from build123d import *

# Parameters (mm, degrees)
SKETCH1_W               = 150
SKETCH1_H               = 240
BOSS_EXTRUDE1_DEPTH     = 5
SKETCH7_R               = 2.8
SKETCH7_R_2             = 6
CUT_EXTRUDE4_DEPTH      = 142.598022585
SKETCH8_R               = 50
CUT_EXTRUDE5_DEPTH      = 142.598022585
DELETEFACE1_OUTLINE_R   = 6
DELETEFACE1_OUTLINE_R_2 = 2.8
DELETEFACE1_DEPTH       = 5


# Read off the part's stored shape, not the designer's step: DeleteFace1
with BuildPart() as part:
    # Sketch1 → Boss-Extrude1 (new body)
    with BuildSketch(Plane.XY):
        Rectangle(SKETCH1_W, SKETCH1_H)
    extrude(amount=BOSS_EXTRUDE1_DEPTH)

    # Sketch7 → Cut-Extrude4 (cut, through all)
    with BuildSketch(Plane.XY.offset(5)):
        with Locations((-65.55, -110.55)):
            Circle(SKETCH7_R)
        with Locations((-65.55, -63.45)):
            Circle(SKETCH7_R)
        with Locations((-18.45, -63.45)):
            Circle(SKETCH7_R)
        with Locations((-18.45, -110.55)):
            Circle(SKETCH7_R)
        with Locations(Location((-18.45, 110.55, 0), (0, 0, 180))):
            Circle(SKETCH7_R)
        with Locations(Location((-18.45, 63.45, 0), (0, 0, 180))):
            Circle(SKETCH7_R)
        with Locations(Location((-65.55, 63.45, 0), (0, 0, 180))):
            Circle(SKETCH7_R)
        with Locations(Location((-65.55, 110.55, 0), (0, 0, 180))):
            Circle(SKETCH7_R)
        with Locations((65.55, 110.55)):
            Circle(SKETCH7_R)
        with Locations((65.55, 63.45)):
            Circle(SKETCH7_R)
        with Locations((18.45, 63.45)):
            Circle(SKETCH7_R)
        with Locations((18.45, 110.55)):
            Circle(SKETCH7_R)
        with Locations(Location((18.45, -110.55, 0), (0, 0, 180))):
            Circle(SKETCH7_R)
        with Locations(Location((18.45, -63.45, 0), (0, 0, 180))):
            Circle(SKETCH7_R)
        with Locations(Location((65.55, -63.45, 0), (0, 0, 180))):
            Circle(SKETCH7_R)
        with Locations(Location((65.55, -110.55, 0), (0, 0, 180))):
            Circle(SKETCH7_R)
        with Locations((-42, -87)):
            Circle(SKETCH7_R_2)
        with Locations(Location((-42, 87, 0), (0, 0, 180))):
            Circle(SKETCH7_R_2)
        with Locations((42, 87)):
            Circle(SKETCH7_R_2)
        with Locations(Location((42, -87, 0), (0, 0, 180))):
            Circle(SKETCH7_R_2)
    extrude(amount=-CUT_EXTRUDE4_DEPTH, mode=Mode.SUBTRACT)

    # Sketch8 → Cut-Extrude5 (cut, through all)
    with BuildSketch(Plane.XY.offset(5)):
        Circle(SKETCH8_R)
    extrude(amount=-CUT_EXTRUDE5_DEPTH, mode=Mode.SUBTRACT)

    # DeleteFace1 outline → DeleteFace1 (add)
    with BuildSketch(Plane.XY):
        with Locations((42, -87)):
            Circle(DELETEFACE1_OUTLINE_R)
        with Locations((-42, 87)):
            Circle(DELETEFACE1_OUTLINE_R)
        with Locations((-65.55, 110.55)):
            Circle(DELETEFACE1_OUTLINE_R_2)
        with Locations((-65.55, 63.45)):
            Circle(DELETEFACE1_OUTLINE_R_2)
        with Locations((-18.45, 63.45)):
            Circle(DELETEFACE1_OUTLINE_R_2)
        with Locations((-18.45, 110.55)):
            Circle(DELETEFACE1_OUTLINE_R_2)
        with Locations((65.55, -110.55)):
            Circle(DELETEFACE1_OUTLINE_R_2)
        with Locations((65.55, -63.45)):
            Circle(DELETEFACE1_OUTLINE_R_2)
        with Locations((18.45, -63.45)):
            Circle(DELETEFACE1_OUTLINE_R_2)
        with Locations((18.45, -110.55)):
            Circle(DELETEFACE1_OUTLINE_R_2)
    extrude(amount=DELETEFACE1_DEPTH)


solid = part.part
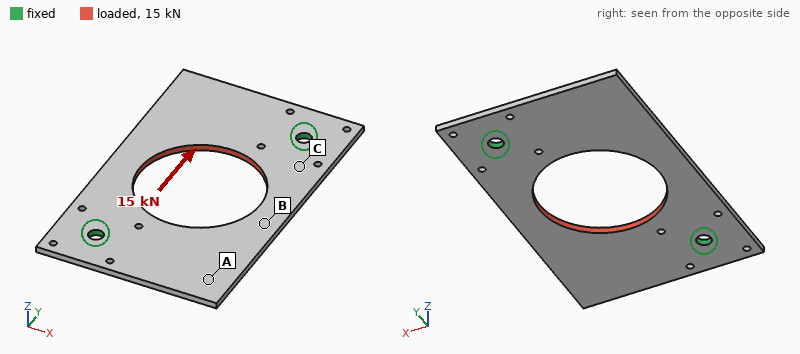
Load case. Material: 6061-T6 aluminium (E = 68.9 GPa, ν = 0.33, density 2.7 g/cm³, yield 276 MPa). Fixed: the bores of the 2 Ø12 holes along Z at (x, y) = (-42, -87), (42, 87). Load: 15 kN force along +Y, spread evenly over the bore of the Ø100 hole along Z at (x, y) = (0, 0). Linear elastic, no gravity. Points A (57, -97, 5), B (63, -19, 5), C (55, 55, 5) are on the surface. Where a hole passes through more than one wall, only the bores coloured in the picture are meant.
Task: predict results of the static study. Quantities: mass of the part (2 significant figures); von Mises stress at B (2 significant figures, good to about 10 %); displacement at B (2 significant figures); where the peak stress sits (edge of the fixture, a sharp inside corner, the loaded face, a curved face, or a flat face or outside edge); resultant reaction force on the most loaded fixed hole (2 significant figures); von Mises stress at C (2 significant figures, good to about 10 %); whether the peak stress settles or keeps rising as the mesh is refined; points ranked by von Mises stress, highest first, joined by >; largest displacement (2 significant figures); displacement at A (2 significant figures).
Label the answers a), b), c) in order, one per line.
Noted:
a) 370 g
b) 14 MPa
c) 37 µm
d) edge of the fixture
e) 7.5 kN
f) 28 MPa
g) keeps rising
h) C > B > A
i) 49 µm
j) 43 µm
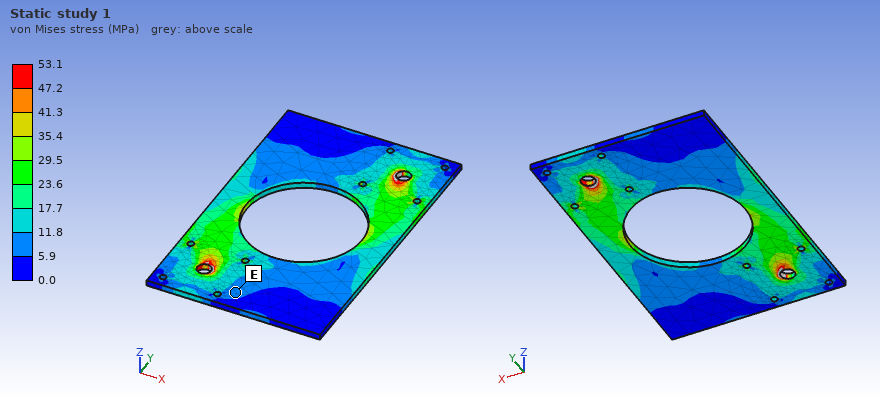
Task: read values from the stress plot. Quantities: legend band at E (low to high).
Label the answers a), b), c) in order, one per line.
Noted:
a) 5.9 to 11.8 MPa
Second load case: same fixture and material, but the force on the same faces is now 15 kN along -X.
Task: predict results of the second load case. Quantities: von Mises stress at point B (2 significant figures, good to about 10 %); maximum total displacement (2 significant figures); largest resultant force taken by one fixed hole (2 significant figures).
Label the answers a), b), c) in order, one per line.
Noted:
a) 26 MPa
b) 71 µm
c) 7.5 kN
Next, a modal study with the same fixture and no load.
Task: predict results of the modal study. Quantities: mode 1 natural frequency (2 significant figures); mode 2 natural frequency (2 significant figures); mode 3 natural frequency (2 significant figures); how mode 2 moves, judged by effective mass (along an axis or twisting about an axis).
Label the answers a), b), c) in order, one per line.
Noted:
a) 320 Hz
b) 360 Hz
c) 780 Hz
d) along Z
